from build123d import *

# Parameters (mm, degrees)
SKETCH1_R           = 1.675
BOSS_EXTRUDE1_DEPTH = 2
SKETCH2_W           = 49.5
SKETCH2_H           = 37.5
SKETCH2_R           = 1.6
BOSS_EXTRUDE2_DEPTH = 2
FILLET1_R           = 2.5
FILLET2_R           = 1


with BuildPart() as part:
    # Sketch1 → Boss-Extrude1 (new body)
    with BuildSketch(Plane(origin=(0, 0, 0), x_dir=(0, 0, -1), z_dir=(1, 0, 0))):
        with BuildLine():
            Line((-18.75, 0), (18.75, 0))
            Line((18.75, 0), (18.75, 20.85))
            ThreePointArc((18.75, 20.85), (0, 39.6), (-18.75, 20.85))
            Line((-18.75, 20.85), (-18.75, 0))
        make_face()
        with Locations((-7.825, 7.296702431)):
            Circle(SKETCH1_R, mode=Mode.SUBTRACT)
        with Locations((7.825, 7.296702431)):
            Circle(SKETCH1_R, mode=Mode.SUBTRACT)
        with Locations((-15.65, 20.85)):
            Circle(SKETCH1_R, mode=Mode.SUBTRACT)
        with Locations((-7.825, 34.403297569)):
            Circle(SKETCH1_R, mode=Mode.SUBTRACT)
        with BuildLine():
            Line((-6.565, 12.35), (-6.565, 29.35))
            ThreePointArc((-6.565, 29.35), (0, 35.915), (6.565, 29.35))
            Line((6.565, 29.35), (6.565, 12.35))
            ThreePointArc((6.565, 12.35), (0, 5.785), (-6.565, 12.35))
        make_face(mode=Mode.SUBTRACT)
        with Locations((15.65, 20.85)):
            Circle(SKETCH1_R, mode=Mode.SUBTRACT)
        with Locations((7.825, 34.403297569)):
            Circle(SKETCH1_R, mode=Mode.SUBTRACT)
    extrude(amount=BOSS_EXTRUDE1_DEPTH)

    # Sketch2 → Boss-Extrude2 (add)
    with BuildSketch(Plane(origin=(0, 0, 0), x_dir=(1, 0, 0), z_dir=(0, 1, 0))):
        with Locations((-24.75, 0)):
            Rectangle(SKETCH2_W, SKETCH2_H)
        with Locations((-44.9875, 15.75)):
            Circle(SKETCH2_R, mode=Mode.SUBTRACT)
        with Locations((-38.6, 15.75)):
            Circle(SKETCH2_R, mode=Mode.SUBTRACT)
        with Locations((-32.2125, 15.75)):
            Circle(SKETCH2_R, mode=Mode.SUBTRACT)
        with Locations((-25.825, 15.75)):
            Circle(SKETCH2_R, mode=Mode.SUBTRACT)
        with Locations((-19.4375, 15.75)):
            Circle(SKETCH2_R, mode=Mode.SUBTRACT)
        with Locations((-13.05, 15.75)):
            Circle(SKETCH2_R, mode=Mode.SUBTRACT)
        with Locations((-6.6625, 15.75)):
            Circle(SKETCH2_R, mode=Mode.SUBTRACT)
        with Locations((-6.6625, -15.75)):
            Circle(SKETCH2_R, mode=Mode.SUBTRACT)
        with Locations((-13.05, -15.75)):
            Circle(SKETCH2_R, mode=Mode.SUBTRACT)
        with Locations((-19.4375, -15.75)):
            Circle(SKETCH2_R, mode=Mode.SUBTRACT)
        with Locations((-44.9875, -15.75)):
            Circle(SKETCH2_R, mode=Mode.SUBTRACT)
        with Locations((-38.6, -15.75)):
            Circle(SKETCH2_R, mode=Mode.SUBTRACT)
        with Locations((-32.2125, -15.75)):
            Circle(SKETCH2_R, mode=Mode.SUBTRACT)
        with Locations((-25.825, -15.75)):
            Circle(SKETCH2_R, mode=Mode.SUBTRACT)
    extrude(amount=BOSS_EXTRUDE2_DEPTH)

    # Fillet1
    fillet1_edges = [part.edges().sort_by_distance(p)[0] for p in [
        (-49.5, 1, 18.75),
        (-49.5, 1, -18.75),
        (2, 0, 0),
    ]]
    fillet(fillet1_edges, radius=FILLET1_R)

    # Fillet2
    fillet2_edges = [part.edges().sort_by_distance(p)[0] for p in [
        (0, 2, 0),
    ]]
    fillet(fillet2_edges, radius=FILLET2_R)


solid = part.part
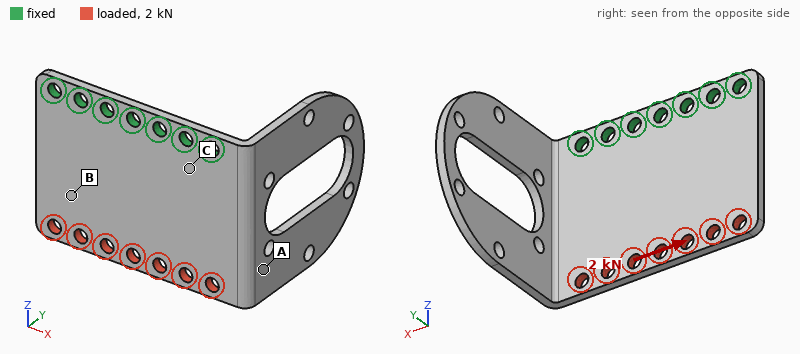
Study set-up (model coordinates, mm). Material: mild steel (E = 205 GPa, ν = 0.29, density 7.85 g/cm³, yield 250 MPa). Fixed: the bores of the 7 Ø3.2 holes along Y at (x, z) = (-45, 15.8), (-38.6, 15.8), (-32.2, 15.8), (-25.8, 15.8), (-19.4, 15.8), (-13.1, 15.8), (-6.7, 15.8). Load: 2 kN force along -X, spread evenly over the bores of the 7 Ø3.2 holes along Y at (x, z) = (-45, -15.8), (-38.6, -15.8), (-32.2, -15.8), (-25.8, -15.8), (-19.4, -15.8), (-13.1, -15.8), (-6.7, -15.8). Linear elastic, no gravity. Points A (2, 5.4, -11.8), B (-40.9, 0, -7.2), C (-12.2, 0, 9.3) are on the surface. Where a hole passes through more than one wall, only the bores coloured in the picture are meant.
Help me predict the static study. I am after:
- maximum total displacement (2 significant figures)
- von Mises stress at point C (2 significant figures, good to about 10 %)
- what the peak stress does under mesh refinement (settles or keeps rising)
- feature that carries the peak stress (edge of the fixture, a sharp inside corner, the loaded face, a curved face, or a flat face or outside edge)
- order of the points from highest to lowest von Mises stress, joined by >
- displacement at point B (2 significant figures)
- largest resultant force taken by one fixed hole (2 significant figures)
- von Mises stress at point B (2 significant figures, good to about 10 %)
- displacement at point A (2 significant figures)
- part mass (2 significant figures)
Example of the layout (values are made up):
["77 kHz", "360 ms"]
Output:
["19 µm", "57 MPa", "keeps rising", "edge of the fixture", "C > B > A", "11 µm", "1.3 kN", "33 MPa", "15 µm", "41 g"]
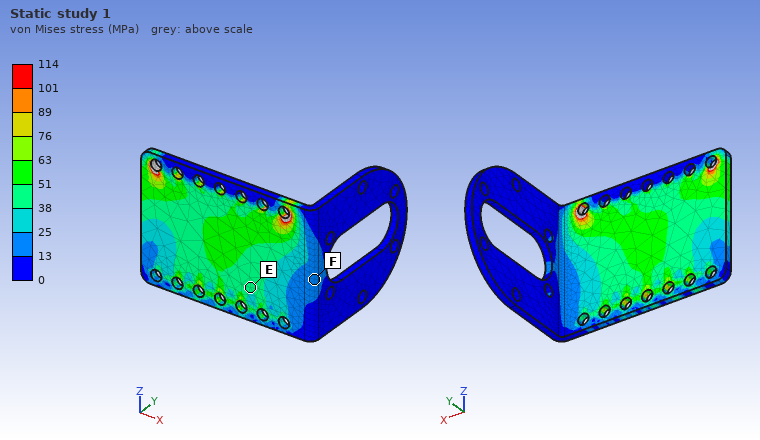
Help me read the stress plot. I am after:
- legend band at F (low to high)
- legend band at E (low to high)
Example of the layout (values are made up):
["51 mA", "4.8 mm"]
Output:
["13 to 25 MPa", "38 to 51 MPa"]
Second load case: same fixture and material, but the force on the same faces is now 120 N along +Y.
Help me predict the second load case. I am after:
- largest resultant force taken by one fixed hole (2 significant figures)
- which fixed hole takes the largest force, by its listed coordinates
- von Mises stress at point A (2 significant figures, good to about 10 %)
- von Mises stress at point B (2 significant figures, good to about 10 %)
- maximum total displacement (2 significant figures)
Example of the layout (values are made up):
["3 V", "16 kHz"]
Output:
["32 N", "(-6.7, 15.8)", "15 MPa", "26 MPa", "0.16 mm"]
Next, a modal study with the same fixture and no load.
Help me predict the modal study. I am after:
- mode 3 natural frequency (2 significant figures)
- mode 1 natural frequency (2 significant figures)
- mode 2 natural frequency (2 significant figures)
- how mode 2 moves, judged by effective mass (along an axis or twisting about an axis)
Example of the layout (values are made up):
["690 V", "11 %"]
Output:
["2200 Hz", "920 Hz", "1200 Hz", "along Y"]
